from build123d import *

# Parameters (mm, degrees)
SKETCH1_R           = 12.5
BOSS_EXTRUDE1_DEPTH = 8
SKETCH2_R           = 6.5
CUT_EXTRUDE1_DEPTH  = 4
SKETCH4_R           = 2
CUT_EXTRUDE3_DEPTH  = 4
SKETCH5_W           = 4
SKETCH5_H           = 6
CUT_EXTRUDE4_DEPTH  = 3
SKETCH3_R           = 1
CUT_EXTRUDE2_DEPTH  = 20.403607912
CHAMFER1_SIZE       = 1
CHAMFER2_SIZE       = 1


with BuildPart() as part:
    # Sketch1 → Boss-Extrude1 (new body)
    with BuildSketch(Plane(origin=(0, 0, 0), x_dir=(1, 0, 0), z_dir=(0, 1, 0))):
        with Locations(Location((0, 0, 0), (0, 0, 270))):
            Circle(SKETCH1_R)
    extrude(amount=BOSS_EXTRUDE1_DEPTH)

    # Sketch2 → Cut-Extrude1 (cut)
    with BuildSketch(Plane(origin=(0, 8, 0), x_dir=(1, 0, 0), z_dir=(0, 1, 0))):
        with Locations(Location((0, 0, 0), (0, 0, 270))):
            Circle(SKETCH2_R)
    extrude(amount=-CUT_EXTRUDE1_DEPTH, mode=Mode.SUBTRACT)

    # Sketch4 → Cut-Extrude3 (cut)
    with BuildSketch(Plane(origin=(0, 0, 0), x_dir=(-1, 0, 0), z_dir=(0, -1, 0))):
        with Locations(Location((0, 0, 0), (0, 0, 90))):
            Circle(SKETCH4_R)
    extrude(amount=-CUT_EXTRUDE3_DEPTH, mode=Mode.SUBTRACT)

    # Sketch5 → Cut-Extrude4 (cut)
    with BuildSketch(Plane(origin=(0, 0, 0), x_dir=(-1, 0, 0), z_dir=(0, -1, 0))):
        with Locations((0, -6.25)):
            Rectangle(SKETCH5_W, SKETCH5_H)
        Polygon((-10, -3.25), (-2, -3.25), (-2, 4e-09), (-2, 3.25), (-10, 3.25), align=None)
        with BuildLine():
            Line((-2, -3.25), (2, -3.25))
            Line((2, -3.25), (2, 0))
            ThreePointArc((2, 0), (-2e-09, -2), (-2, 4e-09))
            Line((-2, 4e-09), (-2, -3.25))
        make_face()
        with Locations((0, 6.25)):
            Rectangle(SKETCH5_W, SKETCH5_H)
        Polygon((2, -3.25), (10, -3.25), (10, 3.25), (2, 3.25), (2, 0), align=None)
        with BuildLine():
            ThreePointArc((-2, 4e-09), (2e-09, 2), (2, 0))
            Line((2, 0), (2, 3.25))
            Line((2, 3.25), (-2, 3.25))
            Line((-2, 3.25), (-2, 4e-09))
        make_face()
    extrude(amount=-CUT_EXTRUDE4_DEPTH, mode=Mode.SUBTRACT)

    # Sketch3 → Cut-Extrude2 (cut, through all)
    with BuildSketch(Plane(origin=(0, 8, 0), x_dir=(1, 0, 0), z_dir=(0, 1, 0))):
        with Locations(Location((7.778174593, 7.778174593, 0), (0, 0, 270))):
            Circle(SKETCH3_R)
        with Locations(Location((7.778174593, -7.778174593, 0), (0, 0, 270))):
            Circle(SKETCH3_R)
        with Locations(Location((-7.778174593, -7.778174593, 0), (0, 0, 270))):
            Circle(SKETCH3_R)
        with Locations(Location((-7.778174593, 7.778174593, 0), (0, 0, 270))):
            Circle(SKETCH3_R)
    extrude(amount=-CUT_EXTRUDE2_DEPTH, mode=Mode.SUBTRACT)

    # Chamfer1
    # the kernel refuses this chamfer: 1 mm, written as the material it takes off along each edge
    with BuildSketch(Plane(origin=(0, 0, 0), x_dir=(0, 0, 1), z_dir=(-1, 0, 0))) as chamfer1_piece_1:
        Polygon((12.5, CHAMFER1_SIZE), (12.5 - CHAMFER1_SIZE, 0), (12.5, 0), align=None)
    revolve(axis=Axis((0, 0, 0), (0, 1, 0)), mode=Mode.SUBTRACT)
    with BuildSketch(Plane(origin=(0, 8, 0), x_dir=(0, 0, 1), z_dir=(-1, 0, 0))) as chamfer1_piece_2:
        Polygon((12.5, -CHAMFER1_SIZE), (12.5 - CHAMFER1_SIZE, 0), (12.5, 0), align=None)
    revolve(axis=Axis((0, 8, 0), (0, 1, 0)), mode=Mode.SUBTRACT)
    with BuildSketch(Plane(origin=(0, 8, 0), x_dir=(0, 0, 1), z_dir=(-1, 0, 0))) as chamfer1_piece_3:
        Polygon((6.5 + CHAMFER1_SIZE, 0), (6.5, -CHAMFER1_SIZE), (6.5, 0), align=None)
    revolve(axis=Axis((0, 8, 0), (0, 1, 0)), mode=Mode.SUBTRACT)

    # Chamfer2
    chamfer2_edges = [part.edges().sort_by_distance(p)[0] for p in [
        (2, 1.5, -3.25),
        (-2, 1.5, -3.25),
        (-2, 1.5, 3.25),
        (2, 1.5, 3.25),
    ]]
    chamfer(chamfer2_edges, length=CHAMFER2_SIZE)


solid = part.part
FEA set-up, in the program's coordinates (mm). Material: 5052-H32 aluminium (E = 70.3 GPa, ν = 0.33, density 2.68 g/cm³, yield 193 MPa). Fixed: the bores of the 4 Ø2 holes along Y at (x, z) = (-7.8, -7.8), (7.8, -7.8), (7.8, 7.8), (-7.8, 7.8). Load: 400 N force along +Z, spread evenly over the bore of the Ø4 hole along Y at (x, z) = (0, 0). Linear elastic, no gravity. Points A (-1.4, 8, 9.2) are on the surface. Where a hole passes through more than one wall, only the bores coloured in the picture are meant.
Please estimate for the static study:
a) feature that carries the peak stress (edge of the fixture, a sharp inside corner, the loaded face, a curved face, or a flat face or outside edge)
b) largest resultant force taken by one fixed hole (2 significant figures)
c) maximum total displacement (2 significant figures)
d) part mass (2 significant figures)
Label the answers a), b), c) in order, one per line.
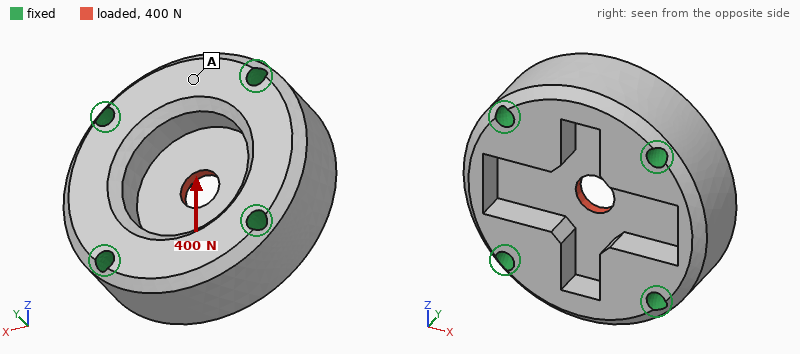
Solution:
a) the loaded face
b) 100 N
c) 2.2 µm
d) 7.1 g
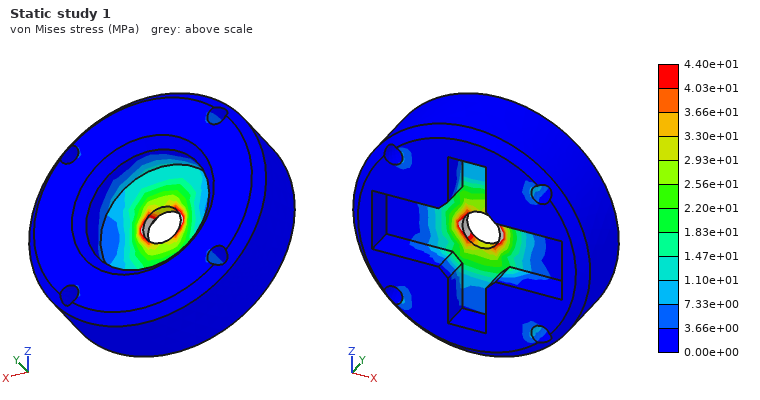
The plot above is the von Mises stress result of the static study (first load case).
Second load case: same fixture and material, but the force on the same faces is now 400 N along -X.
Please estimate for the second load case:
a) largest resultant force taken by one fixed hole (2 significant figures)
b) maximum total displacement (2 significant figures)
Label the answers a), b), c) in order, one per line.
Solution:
a) 100 N
b) 2.2 µm
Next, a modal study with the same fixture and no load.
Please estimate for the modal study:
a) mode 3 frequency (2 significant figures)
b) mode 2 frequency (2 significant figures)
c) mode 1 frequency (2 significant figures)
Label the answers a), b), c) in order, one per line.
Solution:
a) 74 kHz
b) 73 kHz
c) 72 kHz
